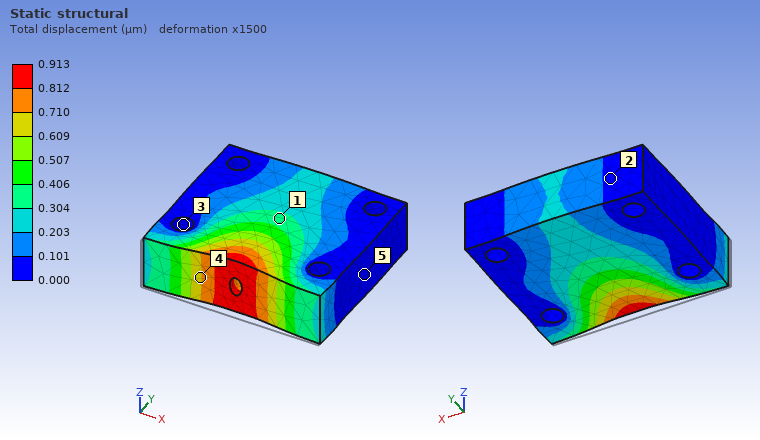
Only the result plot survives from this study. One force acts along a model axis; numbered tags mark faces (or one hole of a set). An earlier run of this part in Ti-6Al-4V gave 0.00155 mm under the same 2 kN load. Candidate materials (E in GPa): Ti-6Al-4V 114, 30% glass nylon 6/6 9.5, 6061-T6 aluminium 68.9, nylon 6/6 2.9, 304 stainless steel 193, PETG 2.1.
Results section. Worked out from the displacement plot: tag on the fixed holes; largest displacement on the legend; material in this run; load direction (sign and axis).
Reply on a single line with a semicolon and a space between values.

3; 0.913 µm; 304 stainless steel; +Y
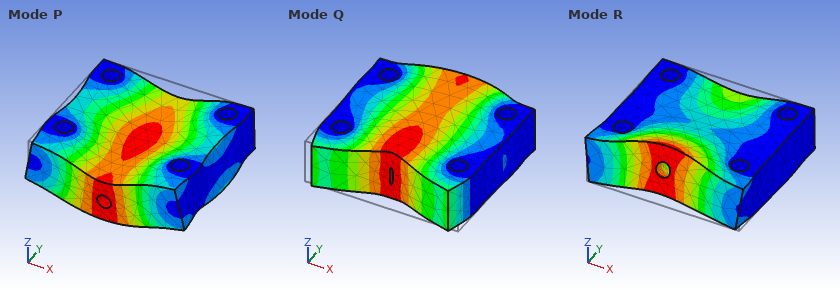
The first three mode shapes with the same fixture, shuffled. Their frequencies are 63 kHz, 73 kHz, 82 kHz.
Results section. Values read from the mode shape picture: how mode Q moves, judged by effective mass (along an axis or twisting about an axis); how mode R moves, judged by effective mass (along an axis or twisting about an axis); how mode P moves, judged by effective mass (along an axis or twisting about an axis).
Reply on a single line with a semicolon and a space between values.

along Y; twisting about X; along Z
